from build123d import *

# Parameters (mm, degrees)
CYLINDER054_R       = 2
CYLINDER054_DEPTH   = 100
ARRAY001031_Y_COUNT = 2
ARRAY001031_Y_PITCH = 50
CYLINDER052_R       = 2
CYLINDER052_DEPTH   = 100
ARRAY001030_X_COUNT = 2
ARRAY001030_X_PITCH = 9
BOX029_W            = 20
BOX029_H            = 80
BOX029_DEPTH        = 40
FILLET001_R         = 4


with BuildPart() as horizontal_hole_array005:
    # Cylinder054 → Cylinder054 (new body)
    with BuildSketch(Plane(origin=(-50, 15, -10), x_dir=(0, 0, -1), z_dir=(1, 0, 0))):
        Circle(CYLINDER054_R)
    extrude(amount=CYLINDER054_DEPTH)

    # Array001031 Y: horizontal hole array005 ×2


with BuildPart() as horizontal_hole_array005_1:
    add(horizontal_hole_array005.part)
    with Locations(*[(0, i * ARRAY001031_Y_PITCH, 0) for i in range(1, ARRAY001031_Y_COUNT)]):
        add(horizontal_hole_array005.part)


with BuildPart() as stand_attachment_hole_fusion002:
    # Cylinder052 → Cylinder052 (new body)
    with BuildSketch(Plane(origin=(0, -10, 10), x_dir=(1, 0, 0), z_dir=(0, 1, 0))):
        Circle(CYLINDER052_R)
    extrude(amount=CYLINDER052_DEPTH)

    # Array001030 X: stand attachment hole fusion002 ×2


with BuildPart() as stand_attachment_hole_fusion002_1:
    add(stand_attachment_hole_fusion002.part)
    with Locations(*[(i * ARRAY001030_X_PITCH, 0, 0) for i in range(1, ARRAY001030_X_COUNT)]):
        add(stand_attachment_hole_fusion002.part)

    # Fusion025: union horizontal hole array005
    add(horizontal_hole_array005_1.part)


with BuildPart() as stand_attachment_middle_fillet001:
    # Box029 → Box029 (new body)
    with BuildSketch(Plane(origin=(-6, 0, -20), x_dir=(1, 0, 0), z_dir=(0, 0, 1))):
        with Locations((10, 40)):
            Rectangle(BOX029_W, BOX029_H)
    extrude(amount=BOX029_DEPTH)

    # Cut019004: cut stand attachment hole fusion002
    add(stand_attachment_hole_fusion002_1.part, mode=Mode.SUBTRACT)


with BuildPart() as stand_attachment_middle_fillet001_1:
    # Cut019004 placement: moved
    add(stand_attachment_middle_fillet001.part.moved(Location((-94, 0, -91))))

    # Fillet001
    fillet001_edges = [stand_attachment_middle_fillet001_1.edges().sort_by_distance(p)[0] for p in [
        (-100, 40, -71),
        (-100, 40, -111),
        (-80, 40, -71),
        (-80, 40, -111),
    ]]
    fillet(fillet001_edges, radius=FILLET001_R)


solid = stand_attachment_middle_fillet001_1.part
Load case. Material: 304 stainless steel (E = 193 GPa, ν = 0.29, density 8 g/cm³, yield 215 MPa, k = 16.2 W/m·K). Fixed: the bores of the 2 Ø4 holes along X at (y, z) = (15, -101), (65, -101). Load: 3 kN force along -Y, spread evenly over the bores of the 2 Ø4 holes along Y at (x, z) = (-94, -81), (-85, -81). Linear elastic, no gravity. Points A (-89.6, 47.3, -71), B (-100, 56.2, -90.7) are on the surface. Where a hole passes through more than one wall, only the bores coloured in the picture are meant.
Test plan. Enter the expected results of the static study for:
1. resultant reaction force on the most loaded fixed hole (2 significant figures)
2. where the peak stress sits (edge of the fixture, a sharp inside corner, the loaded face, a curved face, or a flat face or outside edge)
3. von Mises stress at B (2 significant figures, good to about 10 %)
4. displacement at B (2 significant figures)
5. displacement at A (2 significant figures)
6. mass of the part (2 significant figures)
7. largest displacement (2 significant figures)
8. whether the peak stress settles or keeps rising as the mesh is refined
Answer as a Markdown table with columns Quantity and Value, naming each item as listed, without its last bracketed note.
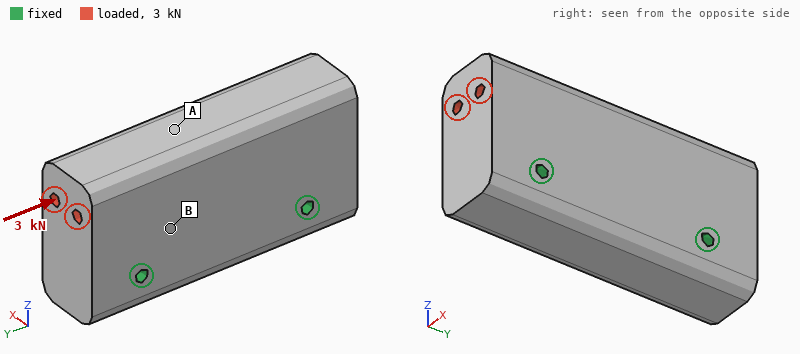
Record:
| Quantity | Value |
|---|---|
| resultant reaction force on the most loaded fixed hole | 1.9 kN |
| where the peak stress sits | edge of the fixture |
| von Mises stress at B | 4.7 MPa |
| displacement at B | 0.50 µm |
| displacement at A | 1.0 µm |
| mass of the part | 480 g |
| largest displacement | 1.4 µm |
| whether the peak stress settles or keeps rising as the mesh is refined | keeps rising |
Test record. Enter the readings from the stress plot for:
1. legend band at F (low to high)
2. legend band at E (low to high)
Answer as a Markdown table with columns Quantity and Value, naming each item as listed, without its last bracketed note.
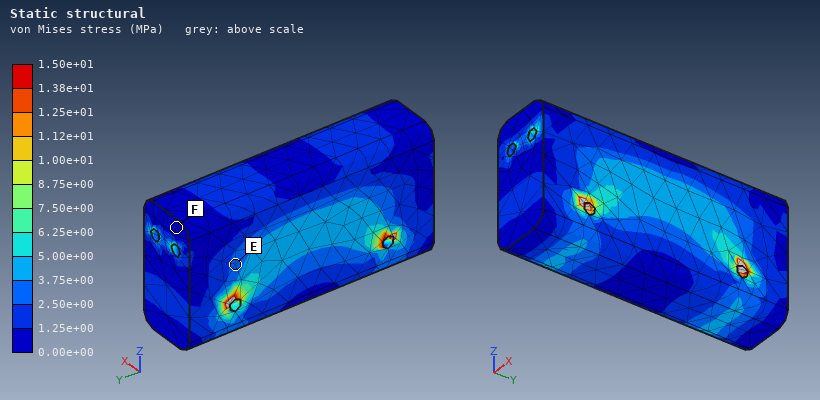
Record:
| Quantity | Value |
|---|---|
| legend band at F | 0.00e+00 to 1.25e+00 MPa |
| legend band at E | 2.50e+00 to 3.75e+00 MPa |
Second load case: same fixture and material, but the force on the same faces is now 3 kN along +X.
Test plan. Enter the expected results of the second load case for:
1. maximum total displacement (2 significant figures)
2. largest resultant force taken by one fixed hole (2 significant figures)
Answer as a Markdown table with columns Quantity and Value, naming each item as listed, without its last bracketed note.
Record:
| Quantity | Value |
|---|---|
| maximum total displacement | 4.7 µm |
| largest resultant force taken by one fixed hole | 1.5 kN |
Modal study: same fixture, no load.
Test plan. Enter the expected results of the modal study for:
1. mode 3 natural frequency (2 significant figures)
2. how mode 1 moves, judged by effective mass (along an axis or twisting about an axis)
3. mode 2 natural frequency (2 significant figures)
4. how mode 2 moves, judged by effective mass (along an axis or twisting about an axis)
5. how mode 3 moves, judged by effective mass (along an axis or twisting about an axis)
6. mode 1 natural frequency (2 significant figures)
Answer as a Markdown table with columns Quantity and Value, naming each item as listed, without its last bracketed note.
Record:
| Quantity | Value |
|---|---|
| mode 3 natural frequency | 17 kHz |
| how mode 1 moves, judged by effective mass | along X |
| mode 2 natural frequency | 14 kHz |
| how mode 2 moves, judged by effective mass | twisting about Z |
| how mode 3 moves, judged by effective mass | along Y |
| mode 1 natural frequency | 9400 Hz |
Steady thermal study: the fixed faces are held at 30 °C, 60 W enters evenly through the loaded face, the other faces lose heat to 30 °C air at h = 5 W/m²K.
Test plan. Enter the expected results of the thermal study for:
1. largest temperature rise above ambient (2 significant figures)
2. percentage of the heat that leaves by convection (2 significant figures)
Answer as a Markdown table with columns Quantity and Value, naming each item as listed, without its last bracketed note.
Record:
| Quantity | Value |
|---|---|
| largest temperature rise above ambient | 72 K |
| percentage of the heat that leaves by convection | 3.7 % |
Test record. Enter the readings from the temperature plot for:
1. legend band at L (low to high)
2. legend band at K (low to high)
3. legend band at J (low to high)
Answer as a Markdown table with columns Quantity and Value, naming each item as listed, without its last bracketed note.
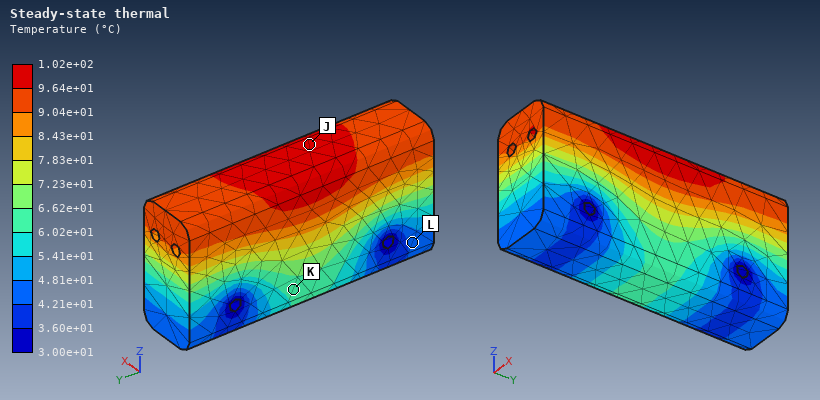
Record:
| Quantity | Value |
|---|---|
| legend band at L | 4.21e+01 to 4.81e+01 °C |
| legend band at K | 6.02e+01 to 6.62e+01 °C |
| legend band at J | 9.64e+01 to 1.02e+02 °C |
